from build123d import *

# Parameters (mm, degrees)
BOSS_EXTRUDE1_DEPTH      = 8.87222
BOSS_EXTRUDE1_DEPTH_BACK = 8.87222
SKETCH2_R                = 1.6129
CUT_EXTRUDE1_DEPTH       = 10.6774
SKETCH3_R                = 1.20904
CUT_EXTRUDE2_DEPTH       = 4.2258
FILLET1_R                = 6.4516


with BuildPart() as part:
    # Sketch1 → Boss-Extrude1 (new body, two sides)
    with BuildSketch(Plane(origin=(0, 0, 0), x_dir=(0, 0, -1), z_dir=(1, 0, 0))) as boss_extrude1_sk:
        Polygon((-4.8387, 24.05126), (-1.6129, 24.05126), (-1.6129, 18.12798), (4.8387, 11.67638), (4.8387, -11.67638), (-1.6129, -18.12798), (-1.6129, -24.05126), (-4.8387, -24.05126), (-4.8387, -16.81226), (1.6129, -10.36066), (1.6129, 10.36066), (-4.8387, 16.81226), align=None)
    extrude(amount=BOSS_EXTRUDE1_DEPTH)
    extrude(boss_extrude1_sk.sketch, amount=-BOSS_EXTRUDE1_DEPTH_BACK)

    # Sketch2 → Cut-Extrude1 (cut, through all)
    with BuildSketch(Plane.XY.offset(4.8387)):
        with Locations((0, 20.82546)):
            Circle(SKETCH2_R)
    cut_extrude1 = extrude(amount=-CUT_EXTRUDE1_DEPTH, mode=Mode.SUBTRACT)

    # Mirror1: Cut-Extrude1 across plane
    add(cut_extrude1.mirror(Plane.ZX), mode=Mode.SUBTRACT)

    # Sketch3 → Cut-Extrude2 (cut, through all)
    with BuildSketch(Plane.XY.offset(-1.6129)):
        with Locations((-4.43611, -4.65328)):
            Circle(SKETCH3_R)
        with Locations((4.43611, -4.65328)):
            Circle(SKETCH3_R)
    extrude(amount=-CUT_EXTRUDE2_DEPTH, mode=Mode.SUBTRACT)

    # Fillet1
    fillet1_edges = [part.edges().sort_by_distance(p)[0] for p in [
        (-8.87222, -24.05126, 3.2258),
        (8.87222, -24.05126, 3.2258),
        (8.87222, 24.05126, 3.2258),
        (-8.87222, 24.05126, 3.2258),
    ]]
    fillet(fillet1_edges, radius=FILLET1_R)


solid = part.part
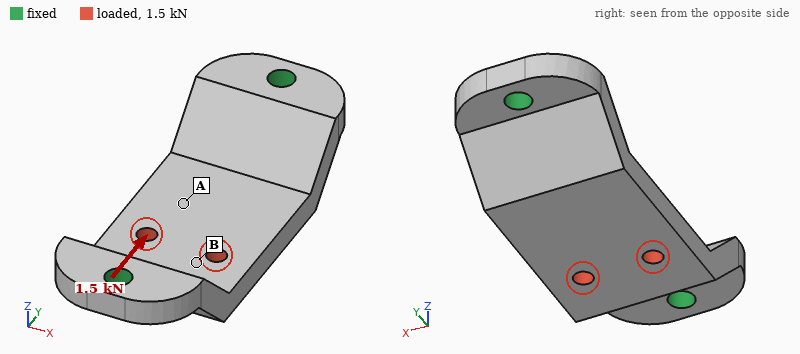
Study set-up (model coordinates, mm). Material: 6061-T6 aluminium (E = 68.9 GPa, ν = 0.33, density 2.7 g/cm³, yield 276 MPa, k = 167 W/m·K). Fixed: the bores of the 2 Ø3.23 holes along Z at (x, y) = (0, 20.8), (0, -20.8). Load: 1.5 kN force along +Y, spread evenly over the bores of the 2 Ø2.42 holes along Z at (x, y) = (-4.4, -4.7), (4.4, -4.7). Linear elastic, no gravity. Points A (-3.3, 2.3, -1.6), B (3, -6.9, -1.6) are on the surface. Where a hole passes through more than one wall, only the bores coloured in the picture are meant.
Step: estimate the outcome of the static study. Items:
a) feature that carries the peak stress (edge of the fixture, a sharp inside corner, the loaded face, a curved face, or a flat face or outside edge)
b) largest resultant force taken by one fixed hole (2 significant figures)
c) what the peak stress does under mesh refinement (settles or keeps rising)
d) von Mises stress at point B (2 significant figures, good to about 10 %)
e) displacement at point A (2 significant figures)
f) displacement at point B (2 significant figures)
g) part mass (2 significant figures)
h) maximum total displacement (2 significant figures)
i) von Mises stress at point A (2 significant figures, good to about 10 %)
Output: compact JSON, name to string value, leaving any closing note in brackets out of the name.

{"feature that carries the peak stress": "a sharp inside corner", "largest resultant force taken by one fixed hole": "780 N", "what the peak stress does under mesh refinement": "keeps rising", "von Mises stress at point B": "55 MPa", "displacement at point A": "20 µm", "displacement at point B": "23 µm", "part mass": "7.7 g", "maximum total displacement": "25 µm", "von Mises stress at point A": "28 MPa"}
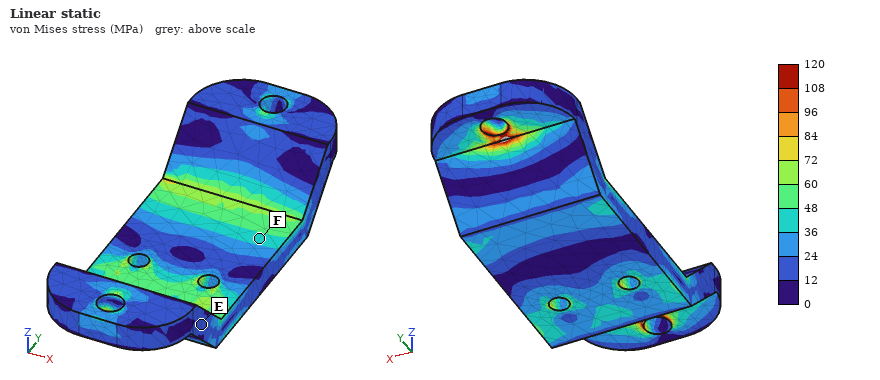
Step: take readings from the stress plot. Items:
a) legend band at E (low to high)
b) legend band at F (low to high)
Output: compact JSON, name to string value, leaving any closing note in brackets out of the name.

{"legend band at E": "12 to 24 MPa", "legend band at F": "36 to 48 MPa"}
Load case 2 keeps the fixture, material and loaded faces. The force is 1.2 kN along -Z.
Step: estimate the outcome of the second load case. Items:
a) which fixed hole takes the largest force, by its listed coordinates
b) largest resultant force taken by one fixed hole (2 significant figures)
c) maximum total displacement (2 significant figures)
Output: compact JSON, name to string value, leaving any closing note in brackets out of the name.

{"which fixed hole takes the largest force, by its listed coordinates": "(0, -20.8)", "largest resultant force taken by one fixed hole": "1.3 kN", "maximum total displacement": "52 µm"}
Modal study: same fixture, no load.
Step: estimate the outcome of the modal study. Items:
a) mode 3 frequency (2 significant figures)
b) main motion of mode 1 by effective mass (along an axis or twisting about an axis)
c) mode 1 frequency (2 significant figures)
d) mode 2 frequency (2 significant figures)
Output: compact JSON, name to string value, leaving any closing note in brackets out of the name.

{"mode 3 frequency": "17 kHz", "main motion of mode 1 by effective mass": "along X", "mode 1 frequency": "10000 Hz", "mode 2 frequency": "17 kHz"}
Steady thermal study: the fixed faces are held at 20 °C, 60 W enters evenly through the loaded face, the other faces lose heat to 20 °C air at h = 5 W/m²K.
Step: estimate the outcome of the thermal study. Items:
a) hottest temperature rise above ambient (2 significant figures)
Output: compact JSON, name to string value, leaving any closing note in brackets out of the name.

{"hottest temperature rise above ambient": "77 K"}
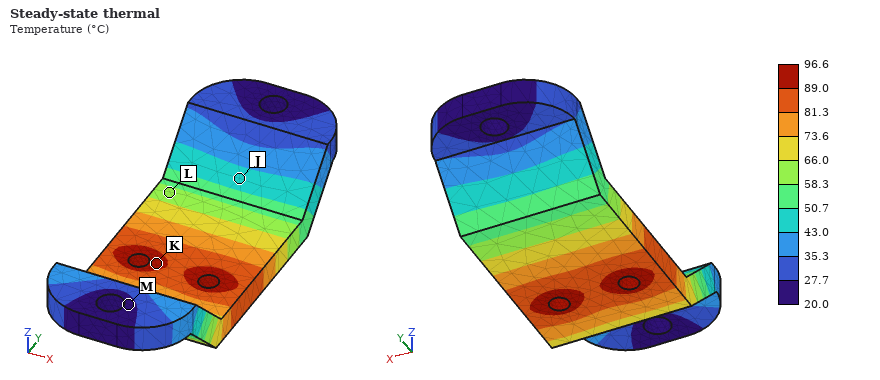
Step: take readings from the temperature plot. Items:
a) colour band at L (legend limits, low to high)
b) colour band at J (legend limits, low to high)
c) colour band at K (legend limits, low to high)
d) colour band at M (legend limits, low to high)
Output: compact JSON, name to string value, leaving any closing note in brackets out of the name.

{"colour band at L": "58.3 to 66.0 °C", "colour band at J": "43.0 to 50.7 °C", "colour band at K": "89.0 to 96.6 °C", "colour band at M": "20.0 to 27.7 °C"}
